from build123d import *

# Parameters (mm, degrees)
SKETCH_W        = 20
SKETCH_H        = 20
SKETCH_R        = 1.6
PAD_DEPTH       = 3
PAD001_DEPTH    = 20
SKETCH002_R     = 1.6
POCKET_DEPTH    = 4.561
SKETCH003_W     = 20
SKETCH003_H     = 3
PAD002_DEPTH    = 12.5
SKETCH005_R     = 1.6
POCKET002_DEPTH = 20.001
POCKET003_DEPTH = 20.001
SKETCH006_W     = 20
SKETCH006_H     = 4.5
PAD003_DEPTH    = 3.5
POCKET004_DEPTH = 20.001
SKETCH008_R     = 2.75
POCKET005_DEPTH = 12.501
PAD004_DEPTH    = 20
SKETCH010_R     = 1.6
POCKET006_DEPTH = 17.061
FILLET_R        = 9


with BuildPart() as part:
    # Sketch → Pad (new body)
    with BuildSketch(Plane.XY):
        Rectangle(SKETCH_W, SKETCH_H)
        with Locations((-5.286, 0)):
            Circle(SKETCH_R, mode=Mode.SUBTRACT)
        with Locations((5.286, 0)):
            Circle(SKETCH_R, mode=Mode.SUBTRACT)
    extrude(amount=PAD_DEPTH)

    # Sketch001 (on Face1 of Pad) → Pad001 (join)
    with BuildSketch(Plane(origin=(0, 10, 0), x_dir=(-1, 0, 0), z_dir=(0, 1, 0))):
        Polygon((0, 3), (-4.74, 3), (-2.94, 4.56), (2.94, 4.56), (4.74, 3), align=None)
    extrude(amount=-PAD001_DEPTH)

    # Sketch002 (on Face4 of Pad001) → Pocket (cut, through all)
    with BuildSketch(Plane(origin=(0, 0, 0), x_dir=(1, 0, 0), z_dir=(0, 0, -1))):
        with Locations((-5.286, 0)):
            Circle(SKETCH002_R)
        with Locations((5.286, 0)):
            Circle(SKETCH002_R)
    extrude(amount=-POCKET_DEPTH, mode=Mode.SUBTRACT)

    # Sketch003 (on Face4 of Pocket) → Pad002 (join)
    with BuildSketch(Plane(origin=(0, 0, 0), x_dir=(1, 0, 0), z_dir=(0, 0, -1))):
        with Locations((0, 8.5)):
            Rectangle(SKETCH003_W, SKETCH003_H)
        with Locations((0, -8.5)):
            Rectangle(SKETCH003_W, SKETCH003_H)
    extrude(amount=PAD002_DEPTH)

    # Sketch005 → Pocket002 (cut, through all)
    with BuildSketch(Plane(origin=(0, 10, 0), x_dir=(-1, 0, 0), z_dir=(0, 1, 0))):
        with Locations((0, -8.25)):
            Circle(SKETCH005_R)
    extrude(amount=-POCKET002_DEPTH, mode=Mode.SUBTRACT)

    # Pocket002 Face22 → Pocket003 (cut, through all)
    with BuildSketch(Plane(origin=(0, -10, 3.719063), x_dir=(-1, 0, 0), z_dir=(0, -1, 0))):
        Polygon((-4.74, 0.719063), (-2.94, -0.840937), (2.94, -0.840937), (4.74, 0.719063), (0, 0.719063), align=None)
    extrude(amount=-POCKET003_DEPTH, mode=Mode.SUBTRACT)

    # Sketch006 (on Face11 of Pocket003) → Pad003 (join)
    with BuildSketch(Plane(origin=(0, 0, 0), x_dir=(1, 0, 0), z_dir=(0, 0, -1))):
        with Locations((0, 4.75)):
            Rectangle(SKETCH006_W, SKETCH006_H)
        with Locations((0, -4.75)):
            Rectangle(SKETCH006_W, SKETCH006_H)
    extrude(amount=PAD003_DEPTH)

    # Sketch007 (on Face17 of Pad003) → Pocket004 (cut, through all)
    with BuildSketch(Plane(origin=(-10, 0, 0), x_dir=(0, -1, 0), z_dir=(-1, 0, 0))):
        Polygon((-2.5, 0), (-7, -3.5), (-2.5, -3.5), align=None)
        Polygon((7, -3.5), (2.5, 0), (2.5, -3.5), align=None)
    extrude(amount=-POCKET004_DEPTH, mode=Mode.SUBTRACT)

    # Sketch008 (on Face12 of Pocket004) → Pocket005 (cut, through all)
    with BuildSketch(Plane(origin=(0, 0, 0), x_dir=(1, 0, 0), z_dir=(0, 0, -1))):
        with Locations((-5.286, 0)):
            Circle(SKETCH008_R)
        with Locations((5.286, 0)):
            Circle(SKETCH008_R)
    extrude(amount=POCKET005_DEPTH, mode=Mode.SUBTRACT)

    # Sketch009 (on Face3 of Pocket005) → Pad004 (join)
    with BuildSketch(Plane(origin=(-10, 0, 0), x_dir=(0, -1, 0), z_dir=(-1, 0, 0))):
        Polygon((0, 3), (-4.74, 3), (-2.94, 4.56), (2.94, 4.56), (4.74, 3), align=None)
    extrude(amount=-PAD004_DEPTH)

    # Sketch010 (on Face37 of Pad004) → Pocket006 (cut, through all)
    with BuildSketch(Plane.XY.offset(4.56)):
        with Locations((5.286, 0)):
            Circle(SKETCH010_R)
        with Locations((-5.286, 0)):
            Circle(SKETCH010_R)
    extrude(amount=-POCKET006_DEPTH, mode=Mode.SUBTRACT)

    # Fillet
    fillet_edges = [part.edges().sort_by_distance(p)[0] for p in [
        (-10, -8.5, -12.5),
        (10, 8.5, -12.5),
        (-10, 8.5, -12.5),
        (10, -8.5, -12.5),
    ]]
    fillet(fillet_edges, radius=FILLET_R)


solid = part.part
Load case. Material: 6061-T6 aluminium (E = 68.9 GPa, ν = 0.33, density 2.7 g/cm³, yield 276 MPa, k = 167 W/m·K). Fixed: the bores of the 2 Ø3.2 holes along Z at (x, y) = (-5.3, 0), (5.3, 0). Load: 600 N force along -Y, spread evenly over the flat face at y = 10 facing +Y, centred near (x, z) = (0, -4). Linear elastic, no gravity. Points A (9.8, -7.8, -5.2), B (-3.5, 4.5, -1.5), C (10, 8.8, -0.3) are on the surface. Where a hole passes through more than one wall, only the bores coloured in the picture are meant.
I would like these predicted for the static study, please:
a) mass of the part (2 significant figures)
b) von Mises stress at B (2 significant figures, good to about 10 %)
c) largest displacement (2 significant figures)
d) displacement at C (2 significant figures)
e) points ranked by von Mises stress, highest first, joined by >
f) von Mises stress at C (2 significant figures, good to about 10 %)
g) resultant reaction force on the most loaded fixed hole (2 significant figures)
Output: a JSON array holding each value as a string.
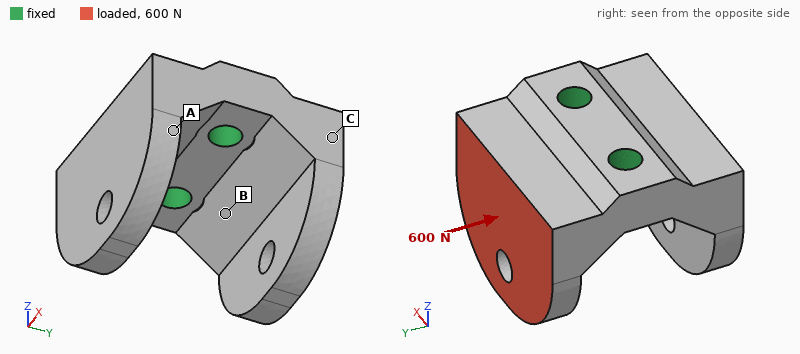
["7.9 g", "39 MPa", "54 µm", "13 µm", "B > C > A", "20 MPa", "300 N"]
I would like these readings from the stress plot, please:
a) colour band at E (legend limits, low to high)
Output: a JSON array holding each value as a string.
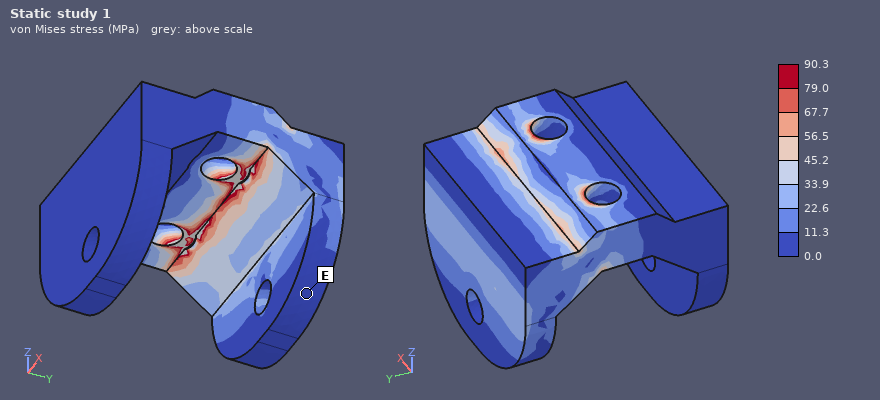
["0.0 to 11.3 MPa"]
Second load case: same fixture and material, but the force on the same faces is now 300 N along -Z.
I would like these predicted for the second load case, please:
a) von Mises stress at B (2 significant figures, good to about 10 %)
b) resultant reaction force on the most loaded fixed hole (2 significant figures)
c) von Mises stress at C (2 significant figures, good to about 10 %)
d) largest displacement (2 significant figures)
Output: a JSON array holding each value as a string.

["14 MPa", "150 N", "9.0 MPa", "27 µm"]
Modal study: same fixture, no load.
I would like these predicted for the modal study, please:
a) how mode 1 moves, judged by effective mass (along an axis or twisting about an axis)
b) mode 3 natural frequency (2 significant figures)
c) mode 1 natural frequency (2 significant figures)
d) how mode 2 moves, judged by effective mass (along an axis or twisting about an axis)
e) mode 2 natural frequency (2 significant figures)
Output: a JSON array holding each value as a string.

["along Y", "22 kHz", "13 kHz", "along Z", "14 kHz"]
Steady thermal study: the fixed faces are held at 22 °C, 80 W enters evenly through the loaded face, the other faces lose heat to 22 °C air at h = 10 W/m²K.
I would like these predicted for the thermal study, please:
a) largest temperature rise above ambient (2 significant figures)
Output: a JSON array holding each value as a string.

["74 K"]
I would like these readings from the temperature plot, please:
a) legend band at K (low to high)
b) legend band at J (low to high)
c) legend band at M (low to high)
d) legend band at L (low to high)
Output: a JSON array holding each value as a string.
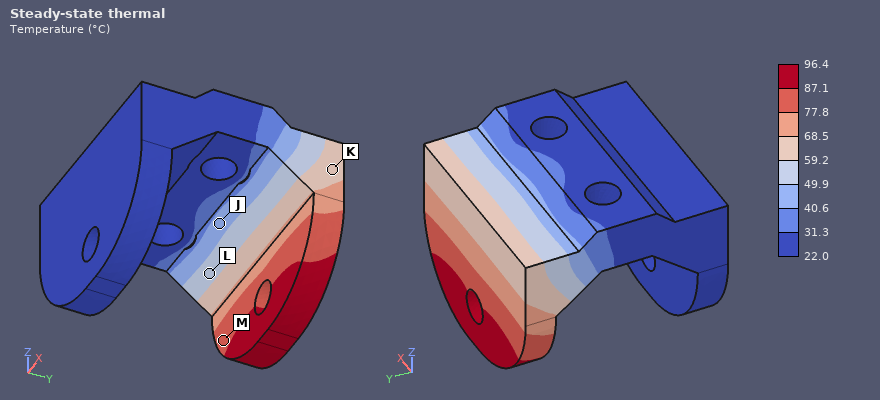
["59.2 to 68.5 °C", "40.6 to 49.9 °C", "77.8 to 87.1 °C", "49.9 to 59.2 °C"]
